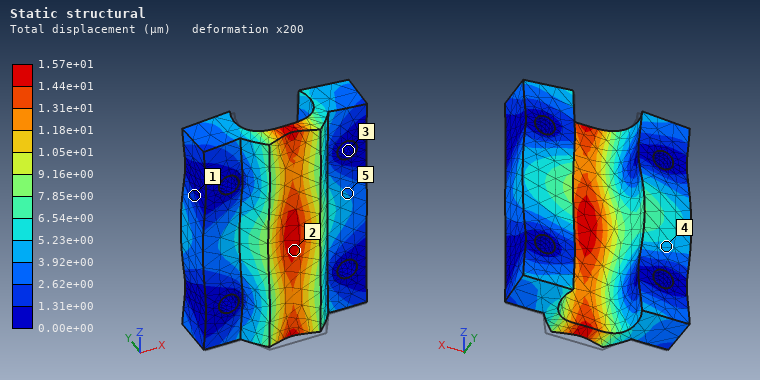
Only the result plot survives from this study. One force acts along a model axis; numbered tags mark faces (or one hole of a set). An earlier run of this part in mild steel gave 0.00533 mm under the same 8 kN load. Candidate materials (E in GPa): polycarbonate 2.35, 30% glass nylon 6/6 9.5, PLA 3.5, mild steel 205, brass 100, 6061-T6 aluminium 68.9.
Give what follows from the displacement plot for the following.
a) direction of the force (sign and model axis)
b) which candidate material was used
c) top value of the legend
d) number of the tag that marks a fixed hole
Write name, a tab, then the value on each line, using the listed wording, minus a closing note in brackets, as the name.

direction of the force	+Y
which candidate material was used	6061-T6 aluminium
top value of the legend	1.57e+01 µm
number of the tag that marks a fixed hole	3
